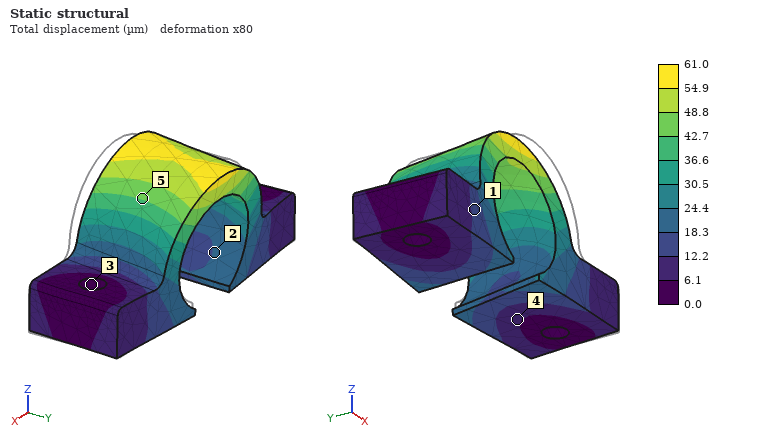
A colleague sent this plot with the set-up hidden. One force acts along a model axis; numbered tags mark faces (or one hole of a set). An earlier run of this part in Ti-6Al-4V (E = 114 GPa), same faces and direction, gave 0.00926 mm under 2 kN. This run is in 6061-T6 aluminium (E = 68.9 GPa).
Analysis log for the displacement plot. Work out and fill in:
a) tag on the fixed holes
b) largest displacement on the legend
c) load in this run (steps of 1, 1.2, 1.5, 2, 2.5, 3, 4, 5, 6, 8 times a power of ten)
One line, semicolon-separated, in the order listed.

3; 61.0 µm; 8 kN
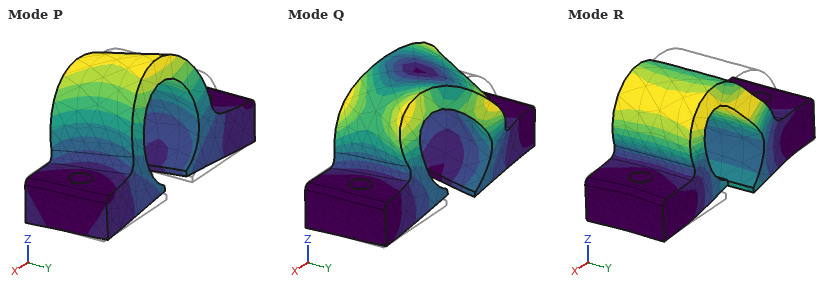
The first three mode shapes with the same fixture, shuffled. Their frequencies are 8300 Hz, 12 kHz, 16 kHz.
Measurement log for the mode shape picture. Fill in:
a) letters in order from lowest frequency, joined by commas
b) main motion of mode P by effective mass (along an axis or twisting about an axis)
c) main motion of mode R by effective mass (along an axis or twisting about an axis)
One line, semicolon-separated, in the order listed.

P, R, Q; along Y; along X
